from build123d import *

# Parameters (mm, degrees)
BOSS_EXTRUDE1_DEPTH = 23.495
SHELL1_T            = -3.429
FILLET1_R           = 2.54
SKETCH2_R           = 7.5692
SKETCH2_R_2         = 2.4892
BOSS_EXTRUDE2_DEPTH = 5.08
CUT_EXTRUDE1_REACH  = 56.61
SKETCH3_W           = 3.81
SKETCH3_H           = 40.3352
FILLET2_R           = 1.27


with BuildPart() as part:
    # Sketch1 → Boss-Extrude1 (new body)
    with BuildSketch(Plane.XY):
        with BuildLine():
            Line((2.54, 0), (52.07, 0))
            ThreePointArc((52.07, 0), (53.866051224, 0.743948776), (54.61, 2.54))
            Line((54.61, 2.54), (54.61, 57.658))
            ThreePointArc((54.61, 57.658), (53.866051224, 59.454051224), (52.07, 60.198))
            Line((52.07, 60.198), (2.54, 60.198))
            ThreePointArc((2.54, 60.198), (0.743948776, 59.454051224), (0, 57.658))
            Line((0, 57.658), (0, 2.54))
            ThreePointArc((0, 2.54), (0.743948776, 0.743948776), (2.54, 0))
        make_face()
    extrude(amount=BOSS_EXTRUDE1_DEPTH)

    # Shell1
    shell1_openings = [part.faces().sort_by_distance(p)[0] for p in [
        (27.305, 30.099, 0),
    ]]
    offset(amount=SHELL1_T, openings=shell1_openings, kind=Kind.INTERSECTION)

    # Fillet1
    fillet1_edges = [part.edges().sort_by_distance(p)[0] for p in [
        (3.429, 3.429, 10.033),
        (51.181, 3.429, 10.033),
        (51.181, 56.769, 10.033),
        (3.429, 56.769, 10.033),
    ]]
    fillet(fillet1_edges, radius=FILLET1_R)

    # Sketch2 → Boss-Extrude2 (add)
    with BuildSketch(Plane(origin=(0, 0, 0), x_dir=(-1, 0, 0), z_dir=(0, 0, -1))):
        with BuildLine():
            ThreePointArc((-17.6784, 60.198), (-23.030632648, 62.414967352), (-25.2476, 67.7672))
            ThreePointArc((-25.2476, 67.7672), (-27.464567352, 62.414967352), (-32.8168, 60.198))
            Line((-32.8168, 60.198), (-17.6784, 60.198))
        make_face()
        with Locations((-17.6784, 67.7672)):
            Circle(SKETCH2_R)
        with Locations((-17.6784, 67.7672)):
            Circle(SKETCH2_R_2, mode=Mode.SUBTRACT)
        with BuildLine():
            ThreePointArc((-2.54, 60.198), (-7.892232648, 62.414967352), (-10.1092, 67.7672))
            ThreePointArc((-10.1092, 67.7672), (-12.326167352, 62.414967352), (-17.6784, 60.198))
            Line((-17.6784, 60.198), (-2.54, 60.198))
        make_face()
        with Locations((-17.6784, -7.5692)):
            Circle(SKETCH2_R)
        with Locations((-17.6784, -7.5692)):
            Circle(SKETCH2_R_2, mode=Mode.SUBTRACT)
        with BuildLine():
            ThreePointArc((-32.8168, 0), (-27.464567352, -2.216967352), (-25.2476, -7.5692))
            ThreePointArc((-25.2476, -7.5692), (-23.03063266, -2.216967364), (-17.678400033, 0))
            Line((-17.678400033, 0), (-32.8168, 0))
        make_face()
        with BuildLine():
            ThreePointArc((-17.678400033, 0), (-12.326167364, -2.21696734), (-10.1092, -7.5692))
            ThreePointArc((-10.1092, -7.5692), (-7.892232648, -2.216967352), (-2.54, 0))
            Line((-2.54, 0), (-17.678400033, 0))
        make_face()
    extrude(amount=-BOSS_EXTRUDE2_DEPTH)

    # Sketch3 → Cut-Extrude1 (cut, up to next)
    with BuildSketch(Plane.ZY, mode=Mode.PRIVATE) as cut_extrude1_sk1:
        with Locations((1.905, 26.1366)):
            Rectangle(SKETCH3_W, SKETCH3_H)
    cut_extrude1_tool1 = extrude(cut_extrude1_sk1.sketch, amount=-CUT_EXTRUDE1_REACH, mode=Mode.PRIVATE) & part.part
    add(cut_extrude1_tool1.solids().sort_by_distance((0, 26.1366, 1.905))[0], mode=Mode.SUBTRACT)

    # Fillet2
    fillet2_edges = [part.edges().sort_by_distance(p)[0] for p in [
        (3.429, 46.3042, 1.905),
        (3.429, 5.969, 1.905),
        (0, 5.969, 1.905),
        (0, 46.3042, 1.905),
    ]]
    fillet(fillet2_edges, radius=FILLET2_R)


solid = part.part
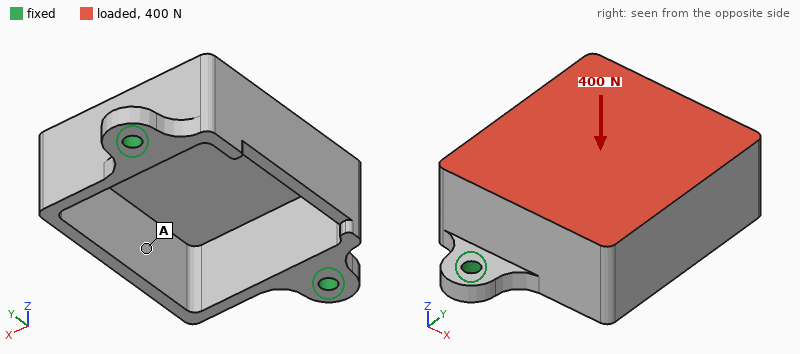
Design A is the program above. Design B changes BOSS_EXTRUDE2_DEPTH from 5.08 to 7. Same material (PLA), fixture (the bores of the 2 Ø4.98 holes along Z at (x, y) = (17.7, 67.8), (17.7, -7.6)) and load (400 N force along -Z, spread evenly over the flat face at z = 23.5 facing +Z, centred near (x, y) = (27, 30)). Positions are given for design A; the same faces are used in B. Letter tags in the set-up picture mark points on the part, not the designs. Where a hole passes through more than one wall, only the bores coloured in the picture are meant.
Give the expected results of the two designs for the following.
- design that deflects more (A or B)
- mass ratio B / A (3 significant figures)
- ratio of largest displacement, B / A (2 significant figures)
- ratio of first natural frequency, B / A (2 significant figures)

A
1.03
0.55
1.4
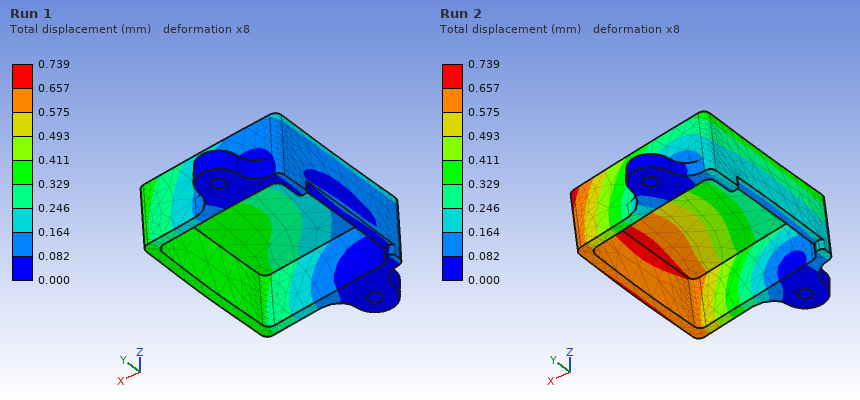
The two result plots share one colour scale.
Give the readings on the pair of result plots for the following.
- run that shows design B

Run 1
